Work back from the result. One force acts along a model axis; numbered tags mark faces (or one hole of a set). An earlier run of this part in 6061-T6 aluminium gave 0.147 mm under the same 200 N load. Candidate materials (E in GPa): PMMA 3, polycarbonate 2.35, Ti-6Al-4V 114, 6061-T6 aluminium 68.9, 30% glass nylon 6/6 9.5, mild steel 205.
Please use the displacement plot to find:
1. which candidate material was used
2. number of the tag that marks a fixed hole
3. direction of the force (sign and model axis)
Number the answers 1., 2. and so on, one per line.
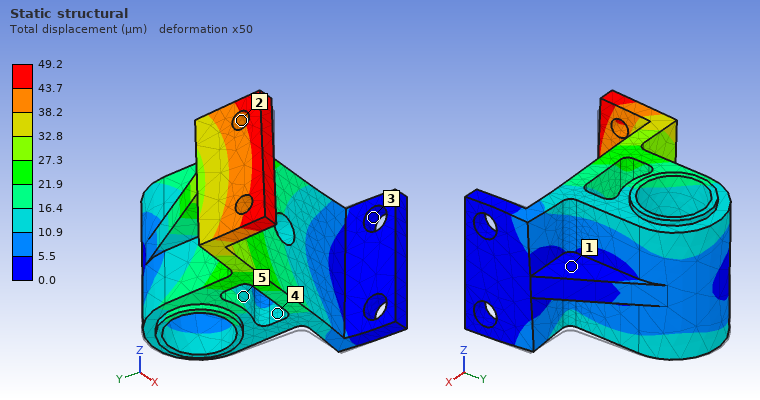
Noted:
1. mild steel
2. 3
3. +Z
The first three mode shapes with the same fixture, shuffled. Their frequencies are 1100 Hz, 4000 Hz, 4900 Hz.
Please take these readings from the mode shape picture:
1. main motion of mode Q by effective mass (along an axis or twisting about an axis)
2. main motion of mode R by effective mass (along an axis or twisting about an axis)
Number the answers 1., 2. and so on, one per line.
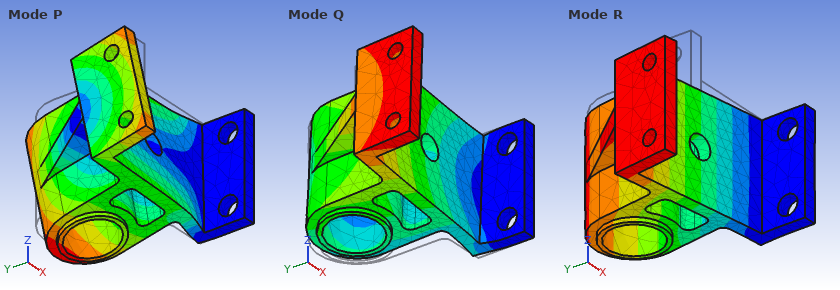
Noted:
1. along Z
2. along Y
